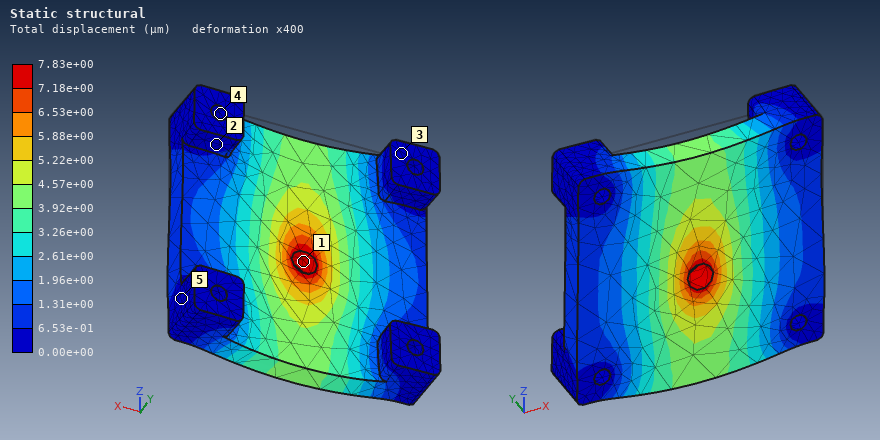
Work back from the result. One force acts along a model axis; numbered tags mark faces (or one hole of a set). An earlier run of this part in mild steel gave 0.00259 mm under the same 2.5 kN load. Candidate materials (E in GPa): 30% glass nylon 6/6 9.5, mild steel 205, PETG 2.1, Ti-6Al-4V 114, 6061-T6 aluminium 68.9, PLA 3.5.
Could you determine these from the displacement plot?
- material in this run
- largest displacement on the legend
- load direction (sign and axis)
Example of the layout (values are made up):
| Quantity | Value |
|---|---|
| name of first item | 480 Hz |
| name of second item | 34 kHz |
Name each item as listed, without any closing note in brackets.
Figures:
| Quantity | Value |
|---|---|
| material in this run | 6061-T6 aluminium |
| largest displacement on the legend | 7.83e+00 µm |
| load direction | -Z |
